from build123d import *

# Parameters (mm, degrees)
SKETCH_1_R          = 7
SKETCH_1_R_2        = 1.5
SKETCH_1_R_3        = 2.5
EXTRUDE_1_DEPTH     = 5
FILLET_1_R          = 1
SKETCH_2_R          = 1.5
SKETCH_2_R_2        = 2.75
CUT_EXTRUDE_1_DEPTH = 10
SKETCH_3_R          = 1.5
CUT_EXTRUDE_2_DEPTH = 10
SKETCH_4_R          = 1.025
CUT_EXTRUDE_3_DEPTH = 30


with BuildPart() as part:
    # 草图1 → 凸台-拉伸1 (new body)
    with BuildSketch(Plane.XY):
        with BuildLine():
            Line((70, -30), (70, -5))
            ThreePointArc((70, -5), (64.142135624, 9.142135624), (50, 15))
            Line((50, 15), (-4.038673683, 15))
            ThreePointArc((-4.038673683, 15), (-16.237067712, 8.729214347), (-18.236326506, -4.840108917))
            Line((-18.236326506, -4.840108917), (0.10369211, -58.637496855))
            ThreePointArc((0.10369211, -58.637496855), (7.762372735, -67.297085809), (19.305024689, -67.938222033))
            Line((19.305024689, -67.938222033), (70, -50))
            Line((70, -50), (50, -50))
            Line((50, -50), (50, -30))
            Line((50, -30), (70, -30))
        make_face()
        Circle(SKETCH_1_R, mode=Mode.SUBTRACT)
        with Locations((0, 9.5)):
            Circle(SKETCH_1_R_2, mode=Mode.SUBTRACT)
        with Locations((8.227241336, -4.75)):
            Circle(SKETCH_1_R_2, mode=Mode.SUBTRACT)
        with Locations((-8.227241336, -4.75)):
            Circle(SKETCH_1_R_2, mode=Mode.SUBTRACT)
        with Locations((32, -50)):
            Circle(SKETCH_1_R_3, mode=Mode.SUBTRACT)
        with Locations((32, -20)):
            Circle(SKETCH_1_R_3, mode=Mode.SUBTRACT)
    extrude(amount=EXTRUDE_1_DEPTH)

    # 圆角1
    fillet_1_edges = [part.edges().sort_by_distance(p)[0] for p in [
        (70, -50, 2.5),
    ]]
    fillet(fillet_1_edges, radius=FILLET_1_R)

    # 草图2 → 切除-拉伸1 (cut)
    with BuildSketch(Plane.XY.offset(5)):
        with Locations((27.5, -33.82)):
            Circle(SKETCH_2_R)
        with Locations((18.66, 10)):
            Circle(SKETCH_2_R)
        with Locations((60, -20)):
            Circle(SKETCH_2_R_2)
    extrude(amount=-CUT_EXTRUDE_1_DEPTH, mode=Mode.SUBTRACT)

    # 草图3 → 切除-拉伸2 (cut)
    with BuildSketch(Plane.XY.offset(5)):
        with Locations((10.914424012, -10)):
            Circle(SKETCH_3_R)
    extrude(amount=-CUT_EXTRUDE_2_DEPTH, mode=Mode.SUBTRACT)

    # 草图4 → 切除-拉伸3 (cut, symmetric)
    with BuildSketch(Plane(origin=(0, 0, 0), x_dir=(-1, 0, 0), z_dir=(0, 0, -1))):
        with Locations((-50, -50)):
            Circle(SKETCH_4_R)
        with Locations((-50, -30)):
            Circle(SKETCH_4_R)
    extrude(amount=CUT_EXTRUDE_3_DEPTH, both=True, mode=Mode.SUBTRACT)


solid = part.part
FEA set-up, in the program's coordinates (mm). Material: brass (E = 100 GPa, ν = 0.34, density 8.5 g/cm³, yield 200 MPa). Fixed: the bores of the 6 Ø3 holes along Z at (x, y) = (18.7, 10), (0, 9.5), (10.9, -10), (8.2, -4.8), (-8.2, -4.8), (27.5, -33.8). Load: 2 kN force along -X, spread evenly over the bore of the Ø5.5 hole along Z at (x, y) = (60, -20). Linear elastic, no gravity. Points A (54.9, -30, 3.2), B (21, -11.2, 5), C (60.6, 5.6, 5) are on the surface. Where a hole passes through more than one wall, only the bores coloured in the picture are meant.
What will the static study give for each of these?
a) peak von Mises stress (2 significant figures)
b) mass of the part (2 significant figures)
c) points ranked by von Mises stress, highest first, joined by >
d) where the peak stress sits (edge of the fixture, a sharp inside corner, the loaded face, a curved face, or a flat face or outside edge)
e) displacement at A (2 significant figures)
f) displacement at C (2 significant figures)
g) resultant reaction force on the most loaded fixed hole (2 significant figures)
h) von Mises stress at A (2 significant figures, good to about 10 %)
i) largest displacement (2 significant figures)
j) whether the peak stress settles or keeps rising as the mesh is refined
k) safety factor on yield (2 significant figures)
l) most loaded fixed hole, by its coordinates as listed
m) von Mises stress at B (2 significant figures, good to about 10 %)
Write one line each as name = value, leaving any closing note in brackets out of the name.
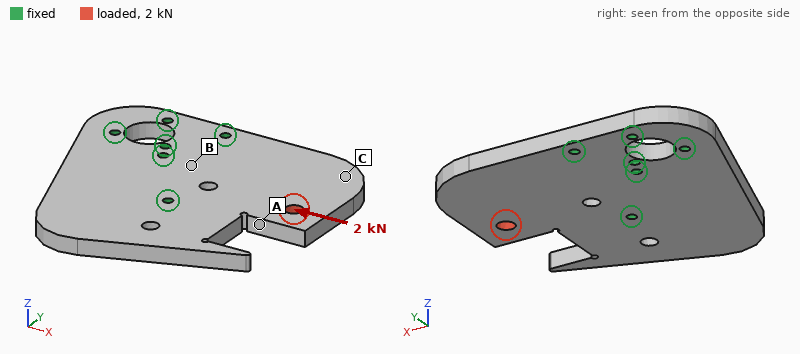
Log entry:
peak von Mises stress = 96 MPa
mass of the part = 230 g
points ranked by von Mises stress, highest first, joined by > = A > B > C
where the peak stress sits = a curved face
displacement at A = 6.1 µm
displacement at C = 1.7 µm
resultant reaction force on the most loaded fixed hole = 1.0 kN
von Mises stress at A = 12 MPa
largest displacement = 8.1 µm
whether the peak stress settles or keeps rising as the mesh is refined = settles
safety factor on yield = 2.1
most loaded fixed hole, by its coordinates as listed = (27.5, -33.8)
von Mises stress at B = 8.2 MPa
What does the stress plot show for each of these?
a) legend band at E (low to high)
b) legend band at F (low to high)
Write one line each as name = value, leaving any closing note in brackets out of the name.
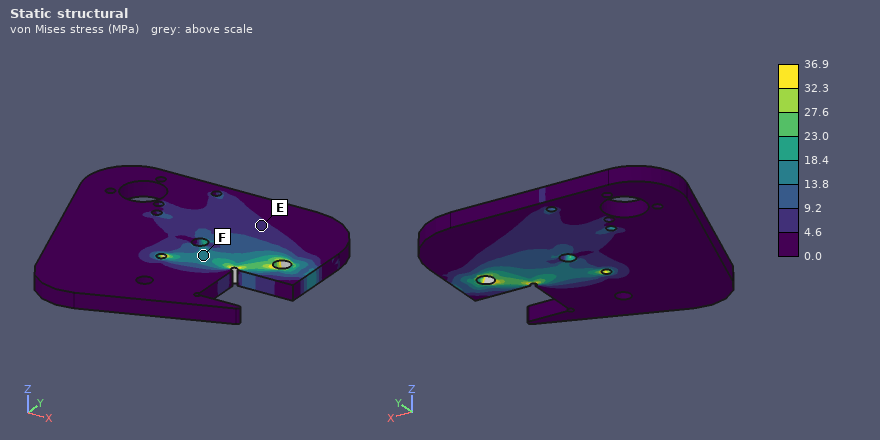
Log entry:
legend band at E = 4.6 to 9.2 MPa
legend band at F = 13.8 to 18.4 MPa
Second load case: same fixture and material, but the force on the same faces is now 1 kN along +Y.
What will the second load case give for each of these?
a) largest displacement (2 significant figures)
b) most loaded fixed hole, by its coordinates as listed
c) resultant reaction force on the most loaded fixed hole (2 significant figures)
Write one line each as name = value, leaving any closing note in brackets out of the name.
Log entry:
largest displacement = 9.3 µm
most loaded fixed hole, by its coordinates as listed = (27.5, -33.8)
resultant reaction force on the most loaded fixed hole = 1.1 kN
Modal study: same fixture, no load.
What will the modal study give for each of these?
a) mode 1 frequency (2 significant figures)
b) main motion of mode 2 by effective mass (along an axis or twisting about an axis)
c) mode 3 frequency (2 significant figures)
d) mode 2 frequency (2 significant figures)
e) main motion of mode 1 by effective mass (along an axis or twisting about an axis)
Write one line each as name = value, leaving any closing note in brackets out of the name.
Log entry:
mode 1 frequency = 1300 Hz
main motion of mode 2 by effective mass = along Z
mode 3 frequency = 2700 Hz
mode 2 frequency = 2100 Hz
main motion of mode 1 by effective mass = along Z
